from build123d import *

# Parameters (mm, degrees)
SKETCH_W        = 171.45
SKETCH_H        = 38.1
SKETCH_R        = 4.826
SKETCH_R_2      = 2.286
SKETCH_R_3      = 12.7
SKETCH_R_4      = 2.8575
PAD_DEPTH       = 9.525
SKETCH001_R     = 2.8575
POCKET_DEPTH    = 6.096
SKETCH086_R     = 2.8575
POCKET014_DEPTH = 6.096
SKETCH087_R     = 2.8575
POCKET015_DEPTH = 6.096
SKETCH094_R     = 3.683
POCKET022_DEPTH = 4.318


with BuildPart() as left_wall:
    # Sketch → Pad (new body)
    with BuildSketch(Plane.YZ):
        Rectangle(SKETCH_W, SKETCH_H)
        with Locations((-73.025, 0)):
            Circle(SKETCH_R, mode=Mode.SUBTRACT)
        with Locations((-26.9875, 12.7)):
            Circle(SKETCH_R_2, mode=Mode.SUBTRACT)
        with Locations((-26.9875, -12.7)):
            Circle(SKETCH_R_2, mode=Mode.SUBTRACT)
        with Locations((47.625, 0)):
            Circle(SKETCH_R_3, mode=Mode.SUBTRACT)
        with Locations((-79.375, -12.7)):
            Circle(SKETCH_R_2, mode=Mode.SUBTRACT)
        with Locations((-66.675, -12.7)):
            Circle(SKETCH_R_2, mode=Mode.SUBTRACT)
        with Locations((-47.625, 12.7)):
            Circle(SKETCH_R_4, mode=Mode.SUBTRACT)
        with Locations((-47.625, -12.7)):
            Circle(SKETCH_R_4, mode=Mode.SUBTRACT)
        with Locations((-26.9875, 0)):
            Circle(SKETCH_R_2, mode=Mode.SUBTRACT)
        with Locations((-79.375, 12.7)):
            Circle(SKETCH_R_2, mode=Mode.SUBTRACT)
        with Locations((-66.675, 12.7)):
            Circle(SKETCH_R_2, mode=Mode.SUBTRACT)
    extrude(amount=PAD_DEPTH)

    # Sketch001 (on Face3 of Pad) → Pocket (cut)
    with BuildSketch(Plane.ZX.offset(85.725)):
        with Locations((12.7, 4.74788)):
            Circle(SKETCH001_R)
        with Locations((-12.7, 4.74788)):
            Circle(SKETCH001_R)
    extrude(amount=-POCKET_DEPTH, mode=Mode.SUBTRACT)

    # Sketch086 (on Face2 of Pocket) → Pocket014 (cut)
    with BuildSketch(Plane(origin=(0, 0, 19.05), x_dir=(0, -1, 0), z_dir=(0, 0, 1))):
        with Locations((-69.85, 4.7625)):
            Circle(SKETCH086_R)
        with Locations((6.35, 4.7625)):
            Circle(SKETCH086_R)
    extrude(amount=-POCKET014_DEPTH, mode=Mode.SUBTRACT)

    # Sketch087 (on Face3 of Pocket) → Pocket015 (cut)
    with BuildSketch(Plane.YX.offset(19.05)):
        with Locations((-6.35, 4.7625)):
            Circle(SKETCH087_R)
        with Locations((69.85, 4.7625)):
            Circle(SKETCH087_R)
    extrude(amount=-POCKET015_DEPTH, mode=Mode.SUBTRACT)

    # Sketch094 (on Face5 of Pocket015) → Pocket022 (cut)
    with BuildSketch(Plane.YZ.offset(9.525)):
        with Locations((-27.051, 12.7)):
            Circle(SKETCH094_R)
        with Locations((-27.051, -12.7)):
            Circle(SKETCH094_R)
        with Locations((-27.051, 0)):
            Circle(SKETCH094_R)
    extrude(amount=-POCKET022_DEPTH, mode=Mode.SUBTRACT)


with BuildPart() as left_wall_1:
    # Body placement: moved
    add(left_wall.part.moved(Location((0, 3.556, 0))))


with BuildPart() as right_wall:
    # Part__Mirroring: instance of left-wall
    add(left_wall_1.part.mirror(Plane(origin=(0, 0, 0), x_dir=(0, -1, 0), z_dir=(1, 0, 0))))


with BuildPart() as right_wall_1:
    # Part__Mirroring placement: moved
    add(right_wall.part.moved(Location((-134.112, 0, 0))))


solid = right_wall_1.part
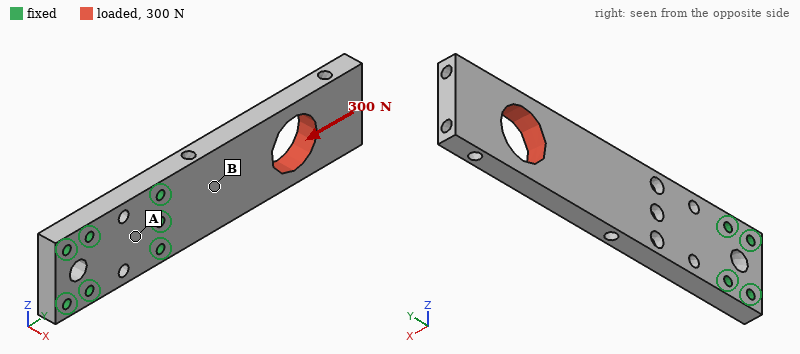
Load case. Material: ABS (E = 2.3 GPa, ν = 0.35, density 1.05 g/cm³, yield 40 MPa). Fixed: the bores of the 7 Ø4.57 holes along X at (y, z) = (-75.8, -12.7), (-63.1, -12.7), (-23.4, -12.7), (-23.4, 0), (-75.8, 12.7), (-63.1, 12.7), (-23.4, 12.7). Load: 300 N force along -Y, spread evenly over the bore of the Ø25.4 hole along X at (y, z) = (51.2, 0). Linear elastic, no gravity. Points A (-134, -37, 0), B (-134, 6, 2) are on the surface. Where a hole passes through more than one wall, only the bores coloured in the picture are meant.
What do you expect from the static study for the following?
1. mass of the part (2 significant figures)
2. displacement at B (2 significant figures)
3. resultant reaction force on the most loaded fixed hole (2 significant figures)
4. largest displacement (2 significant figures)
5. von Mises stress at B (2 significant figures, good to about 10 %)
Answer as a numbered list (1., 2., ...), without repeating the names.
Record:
1. 57 g
2. 0.025 mm
3. 92 N
4. 0.11 mm
5. 0.84 MPa
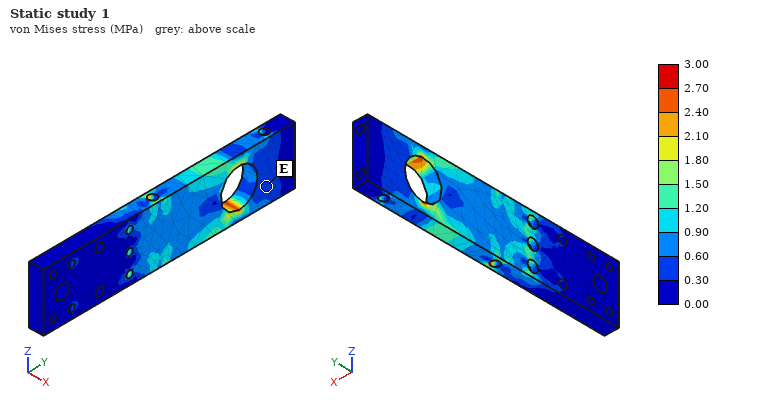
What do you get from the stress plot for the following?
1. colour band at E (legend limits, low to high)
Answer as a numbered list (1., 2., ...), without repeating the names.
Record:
1. 0.30 to 0.60 MPa
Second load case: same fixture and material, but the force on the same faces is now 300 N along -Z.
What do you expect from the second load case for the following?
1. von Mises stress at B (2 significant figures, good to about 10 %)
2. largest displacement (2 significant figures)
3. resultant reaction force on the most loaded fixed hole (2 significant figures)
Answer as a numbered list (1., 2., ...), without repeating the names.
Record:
1. 3.0 MPa
2. 1.2 mm
3. 710 N
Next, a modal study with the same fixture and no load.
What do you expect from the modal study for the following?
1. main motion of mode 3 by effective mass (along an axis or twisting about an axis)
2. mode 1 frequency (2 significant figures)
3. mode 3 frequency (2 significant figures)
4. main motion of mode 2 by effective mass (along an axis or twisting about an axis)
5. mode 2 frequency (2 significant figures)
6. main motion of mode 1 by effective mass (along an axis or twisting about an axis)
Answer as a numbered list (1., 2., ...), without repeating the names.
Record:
1. twisting about Y
2. 180 Hz
3. 900 Hz
4. along Z
5. 610 Hz
6. along X
